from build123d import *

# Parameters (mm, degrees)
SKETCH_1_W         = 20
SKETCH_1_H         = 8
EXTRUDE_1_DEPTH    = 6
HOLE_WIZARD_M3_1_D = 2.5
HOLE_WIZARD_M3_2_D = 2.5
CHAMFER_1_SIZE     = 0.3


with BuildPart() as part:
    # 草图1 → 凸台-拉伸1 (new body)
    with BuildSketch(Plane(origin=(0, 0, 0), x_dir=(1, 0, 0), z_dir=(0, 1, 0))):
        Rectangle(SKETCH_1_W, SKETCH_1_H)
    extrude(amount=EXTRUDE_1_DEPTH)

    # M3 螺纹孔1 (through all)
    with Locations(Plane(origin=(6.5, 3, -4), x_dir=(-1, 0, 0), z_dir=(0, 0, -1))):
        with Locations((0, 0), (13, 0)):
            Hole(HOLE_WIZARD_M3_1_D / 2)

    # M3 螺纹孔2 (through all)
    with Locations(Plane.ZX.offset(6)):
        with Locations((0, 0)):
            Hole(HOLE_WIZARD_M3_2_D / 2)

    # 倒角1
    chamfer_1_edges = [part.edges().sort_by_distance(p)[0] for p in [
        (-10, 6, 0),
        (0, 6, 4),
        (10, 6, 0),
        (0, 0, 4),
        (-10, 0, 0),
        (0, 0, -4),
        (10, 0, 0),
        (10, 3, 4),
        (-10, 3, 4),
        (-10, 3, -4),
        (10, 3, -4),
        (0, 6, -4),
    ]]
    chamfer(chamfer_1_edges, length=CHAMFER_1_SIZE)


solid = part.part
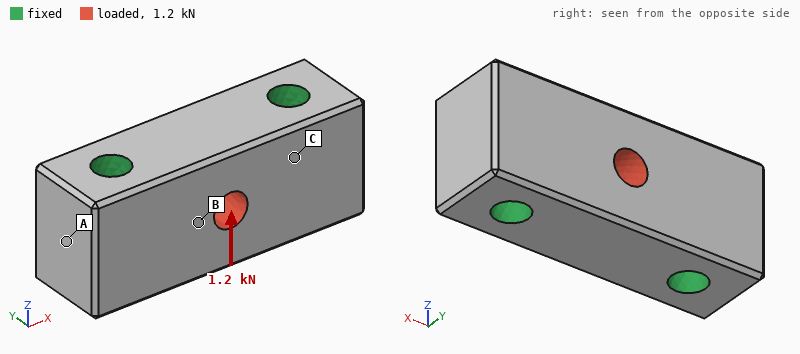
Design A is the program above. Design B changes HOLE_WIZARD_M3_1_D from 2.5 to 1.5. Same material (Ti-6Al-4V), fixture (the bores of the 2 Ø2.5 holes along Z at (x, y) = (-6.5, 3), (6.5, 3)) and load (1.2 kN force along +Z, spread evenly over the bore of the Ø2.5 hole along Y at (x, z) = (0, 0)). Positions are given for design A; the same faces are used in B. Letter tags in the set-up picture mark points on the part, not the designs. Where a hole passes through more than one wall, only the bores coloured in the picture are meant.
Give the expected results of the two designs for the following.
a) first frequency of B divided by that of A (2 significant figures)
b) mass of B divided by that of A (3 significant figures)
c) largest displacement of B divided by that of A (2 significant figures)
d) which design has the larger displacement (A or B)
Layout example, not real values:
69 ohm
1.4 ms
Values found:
0.77
1.06
1.2
B
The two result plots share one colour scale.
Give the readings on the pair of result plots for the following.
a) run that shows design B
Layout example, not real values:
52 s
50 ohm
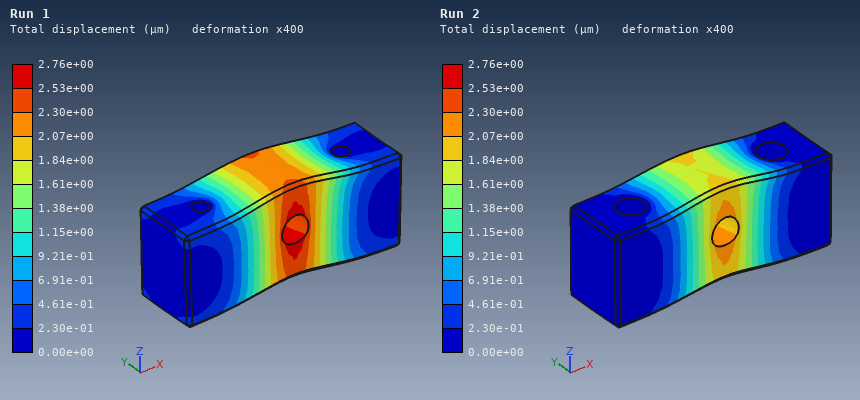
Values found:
Run 1
